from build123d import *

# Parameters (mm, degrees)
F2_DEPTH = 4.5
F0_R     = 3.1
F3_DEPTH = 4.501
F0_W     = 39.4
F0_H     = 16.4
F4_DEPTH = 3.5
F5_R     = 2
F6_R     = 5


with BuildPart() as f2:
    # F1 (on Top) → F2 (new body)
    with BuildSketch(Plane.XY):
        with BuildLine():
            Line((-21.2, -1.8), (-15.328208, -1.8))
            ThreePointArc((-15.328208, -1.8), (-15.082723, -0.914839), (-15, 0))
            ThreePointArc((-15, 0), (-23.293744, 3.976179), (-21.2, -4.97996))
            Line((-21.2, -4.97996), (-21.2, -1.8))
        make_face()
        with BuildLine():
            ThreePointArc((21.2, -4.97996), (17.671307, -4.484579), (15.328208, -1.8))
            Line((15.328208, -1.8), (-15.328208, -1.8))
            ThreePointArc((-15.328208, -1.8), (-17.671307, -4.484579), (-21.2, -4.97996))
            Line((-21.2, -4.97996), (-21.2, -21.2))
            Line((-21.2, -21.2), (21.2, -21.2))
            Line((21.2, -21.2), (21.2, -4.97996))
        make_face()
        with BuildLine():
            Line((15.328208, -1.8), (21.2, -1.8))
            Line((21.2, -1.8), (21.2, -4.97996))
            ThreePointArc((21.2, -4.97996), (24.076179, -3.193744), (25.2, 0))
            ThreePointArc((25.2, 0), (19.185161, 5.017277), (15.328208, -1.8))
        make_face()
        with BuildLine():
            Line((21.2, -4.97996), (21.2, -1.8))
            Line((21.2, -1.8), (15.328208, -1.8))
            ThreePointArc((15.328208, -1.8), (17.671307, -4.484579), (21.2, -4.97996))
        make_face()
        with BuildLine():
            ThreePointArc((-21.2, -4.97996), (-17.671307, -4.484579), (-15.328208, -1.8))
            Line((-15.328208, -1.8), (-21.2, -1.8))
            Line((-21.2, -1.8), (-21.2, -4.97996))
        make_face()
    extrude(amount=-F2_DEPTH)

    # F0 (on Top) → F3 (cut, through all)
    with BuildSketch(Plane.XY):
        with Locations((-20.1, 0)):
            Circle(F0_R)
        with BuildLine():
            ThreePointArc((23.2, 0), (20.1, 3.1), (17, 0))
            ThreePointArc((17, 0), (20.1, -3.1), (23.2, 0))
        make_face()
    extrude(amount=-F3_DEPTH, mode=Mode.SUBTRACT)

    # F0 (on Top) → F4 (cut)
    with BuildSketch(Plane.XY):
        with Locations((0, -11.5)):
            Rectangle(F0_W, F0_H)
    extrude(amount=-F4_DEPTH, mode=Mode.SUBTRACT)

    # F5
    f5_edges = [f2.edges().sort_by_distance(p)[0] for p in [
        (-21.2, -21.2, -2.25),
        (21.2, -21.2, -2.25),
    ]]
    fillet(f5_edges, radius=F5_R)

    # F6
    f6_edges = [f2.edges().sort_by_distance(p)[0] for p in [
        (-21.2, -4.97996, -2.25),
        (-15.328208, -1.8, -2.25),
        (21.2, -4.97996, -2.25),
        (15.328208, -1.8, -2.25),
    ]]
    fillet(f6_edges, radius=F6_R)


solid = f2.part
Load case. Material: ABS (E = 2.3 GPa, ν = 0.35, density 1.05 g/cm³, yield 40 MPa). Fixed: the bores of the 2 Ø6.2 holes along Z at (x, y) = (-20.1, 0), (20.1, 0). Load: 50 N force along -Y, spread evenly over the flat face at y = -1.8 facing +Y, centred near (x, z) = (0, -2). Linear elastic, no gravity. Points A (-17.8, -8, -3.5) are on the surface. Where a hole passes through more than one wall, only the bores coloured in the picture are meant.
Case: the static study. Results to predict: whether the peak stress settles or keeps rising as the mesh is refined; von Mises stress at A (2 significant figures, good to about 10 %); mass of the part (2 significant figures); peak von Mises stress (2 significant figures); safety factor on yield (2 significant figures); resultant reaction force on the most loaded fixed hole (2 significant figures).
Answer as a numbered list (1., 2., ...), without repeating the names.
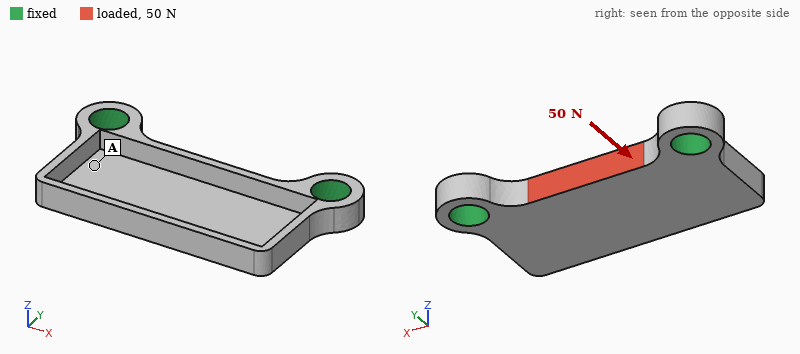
1. settles
2. 1.9 MPa
3. 1.9 g
4. 12 MPa
5. 3.4
6. 30 N
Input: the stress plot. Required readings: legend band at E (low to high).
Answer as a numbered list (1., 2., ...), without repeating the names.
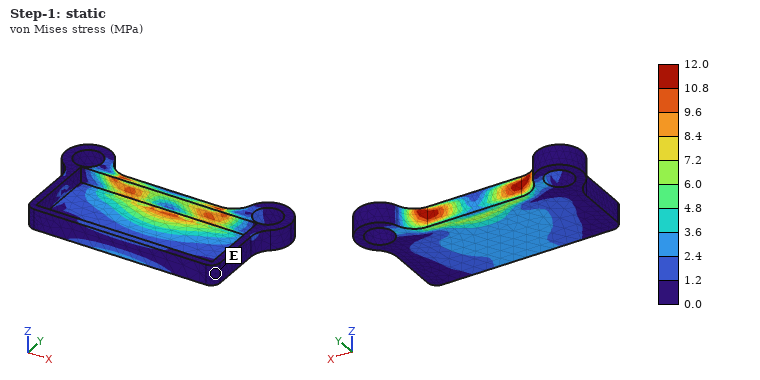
1. 0.0 to 1.2 MPa
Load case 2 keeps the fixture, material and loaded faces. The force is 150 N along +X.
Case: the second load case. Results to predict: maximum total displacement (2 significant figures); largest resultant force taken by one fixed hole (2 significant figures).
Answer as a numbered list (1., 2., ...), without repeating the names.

1. 46 µm
2. 75 N
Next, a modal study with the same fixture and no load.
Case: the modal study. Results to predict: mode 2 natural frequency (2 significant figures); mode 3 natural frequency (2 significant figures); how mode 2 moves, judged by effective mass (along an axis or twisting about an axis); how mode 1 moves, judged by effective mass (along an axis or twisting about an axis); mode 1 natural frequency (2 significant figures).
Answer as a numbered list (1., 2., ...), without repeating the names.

1. 2500 Hz
2. 3400 Hz
3. twisting about Y
4. along Z
5. 1300 Hz
